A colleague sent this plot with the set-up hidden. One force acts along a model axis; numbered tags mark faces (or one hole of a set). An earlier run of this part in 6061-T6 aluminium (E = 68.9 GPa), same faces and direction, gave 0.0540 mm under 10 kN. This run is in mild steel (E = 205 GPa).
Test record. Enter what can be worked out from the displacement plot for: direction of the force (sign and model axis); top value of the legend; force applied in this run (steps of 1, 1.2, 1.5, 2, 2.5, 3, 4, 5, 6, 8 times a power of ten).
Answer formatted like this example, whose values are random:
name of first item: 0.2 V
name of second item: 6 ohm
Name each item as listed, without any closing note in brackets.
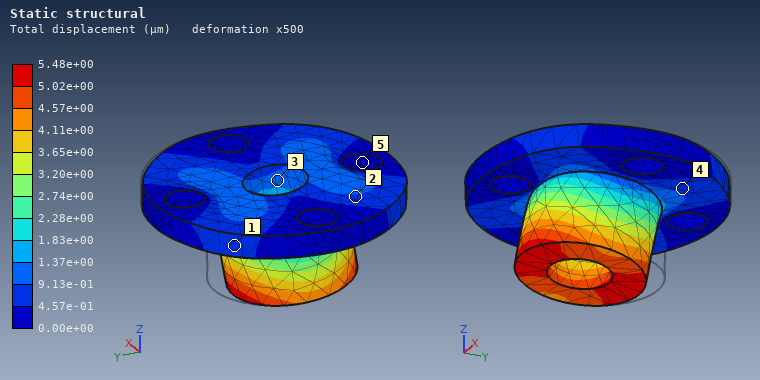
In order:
direction of the force: -Y
top value of the legend: 5.48e+00 µm
force applied in this run: 3 kN
